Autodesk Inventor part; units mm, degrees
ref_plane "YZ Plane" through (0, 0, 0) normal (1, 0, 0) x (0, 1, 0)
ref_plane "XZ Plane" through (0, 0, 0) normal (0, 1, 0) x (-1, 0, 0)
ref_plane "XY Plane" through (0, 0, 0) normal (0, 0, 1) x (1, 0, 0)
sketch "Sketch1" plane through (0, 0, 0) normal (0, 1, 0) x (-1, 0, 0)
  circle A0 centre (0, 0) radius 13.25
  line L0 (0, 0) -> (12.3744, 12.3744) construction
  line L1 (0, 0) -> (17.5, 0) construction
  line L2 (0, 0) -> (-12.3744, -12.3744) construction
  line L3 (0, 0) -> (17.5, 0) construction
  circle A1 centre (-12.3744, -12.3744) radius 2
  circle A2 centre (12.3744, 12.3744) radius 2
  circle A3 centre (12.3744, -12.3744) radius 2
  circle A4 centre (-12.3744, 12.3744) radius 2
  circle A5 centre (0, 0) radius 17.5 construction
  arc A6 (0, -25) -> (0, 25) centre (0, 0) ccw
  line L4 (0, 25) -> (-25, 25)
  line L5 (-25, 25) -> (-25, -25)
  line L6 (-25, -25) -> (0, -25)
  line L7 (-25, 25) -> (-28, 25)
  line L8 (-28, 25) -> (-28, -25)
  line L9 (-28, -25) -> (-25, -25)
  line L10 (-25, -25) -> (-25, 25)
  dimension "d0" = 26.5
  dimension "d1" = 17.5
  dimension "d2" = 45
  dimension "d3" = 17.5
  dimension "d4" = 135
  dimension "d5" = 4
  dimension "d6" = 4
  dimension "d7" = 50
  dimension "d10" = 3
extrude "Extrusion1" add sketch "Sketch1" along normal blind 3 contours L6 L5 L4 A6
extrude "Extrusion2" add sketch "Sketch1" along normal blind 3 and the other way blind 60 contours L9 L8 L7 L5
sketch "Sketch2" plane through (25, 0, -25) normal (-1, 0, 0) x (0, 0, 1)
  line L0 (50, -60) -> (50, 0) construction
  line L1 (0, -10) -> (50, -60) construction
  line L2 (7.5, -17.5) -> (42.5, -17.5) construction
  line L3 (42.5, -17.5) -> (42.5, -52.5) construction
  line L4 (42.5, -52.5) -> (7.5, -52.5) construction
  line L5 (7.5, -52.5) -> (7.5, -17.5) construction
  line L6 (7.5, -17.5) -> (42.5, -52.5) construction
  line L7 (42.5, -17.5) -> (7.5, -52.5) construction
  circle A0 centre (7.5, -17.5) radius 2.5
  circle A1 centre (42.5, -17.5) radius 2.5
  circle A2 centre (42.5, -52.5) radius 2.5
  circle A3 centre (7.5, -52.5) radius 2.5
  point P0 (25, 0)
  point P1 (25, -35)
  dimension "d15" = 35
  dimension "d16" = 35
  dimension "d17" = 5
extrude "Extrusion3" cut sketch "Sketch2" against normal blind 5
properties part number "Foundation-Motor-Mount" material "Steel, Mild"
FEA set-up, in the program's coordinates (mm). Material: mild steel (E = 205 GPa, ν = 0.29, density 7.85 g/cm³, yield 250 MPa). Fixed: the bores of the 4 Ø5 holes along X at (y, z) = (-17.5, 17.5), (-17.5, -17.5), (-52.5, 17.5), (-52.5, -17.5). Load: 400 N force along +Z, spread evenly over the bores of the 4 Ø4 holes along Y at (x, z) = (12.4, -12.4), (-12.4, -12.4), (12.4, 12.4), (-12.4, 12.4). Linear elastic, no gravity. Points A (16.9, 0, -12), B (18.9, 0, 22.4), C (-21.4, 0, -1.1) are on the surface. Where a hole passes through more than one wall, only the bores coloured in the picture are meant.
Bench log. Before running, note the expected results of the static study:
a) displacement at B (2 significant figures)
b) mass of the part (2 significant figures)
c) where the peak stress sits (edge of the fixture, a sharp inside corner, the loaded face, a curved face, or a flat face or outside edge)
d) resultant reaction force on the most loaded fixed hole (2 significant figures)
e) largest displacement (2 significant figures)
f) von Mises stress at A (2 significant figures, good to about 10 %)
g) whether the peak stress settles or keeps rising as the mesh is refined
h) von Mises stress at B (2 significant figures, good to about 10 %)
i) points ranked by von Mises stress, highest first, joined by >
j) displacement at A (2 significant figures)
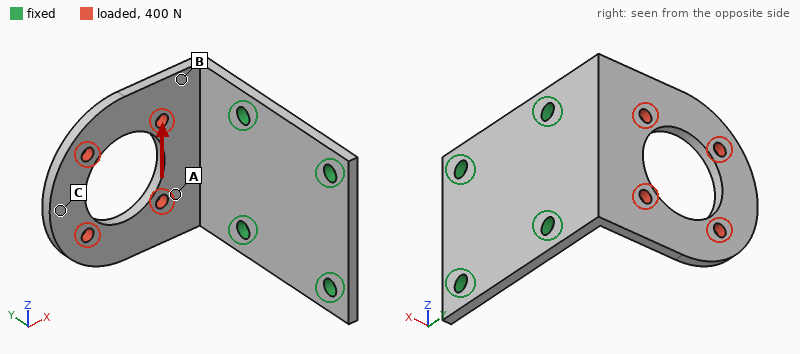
38 µm
110 g
edge of the fixture
400 N
89 µm
26 MPa
keeps rising
39 MPa
B > A > C
26 µm
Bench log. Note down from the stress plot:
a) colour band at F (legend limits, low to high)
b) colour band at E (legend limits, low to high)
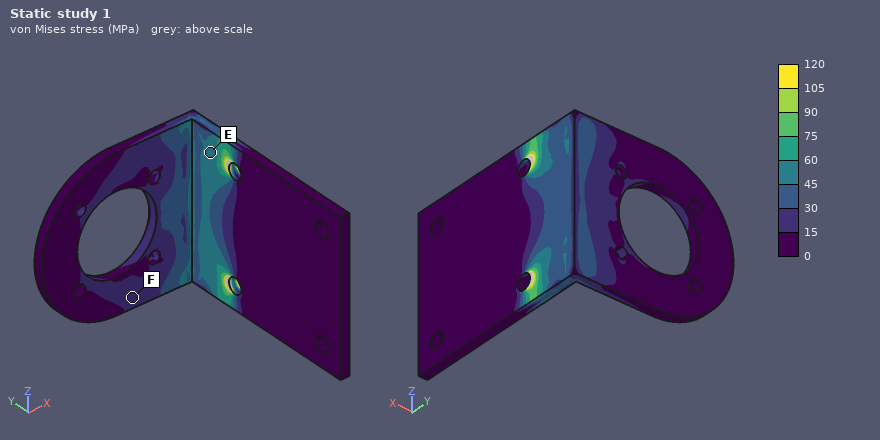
15 to 30 MPa
45 to 60 MPa
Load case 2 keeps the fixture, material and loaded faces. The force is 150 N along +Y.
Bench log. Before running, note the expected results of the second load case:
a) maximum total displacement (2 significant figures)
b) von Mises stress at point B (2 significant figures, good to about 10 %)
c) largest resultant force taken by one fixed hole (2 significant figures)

0.30 mm
42 MPa
65 N
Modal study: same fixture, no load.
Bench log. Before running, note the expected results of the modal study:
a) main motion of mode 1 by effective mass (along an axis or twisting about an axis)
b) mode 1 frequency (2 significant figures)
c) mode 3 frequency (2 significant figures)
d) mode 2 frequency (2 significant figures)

along Y
750 Hz
2700 Hz
1800 Hz
